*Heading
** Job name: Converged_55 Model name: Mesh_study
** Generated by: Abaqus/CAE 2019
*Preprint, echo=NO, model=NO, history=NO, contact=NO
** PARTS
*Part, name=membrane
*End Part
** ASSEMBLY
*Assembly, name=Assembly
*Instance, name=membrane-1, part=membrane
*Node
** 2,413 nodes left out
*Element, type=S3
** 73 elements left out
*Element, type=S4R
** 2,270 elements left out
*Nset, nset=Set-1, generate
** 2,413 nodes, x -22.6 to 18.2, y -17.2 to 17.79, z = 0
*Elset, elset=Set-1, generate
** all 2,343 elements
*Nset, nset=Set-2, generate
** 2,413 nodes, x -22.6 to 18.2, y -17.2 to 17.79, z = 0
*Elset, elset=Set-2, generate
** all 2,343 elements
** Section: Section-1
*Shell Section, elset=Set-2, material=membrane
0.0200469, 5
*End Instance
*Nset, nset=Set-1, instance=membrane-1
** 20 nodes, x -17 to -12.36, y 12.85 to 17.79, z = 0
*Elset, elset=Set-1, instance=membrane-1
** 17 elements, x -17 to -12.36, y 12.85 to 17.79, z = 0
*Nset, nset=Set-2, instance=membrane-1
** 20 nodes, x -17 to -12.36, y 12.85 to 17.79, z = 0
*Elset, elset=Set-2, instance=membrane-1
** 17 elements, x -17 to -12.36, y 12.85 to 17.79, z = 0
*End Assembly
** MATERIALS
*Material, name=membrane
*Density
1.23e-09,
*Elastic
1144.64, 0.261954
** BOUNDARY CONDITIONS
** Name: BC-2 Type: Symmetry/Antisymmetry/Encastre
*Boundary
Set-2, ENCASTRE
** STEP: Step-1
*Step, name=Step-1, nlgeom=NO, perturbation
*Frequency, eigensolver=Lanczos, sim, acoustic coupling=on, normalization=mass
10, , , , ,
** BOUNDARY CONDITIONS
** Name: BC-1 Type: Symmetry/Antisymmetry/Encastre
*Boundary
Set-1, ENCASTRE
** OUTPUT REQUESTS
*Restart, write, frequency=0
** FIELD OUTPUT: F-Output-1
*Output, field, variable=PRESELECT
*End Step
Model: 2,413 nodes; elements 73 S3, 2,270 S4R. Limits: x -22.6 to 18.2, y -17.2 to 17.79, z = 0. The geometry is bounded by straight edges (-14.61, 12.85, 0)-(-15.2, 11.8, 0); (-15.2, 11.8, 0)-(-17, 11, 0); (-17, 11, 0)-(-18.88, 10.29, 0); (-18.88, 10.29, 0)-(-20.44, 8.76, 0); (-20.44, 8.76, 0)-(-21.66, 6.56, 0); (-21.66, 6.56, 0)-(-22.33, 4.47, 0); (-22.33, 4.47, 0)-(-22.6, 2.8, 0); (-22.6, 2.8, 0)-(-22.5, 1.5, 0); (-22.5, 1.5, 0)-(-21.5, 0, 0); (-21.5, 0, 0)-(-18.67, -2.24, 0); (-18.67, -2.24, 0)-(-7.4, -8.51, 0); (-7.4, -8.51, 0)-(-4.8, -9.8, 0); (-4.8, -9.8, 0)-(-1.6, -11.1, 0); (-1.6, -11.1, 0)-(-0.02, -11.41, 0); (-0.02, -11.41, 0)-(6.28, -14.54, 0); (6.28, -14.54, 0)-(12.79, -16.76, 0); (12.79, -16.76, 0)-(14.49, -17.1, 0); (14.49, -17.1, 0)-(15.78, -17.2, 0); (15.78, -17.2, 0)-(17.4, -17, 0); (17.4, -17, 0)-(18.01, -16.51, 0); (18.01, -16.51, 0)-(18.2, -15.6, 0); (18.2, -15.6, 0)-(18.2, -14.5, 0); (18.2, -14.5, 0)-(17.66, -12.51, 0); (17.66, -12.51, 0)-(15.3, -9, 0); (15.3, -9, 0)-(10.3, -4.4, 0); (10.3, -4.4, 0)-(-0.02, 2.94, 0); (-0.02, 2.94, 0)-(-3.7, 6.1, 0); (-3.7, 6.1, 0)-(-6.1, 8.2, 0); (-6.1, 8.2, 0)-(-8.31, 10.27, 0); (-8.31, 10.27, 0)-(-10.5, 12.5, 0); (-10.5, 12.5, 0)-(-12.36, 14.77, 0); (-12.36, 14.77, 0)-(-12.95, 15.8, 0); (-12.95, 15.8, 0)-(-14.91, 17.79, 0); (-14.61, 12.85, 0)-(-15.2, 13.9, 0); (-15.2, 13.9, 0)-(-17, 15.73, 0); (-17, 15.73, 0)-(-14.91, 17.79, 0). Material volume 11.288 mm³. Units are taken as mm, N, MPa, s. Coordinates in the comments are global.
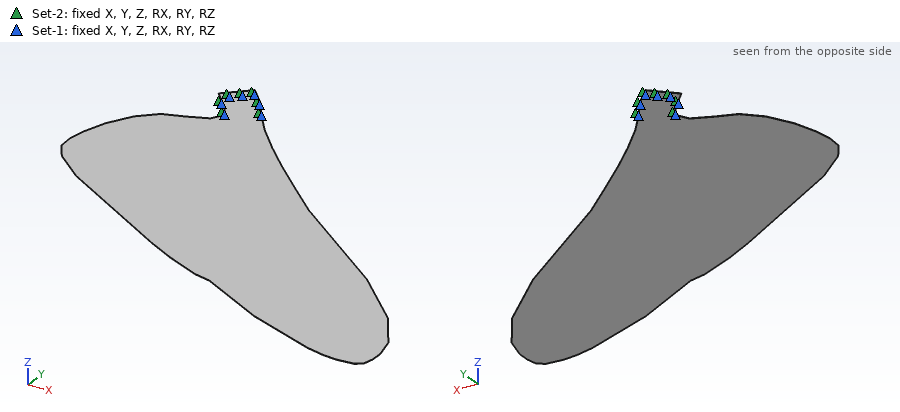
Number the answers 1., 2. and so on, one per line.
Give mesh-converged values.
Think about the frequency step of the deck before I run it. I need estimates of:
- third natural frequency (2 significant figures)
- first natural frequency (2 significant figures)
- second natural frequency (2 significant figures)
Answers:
1. 13 Hz
2. 1.6 Hz
3. 6.7 Hz
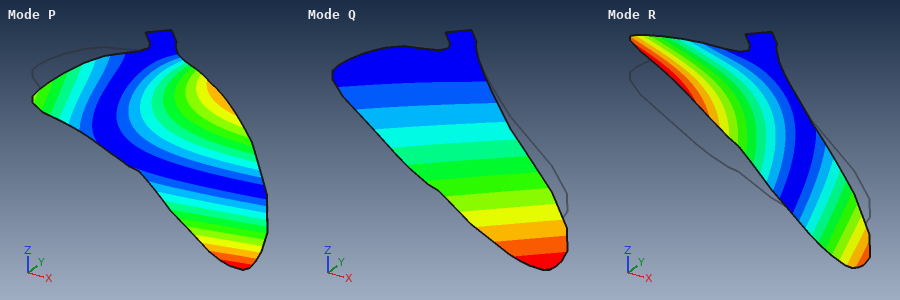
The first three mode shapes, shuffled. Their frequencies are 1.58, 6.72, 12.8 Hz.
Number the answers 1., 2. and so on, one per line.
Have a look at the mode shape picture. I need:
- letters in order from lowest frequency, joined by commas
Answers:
1. Q, R, P
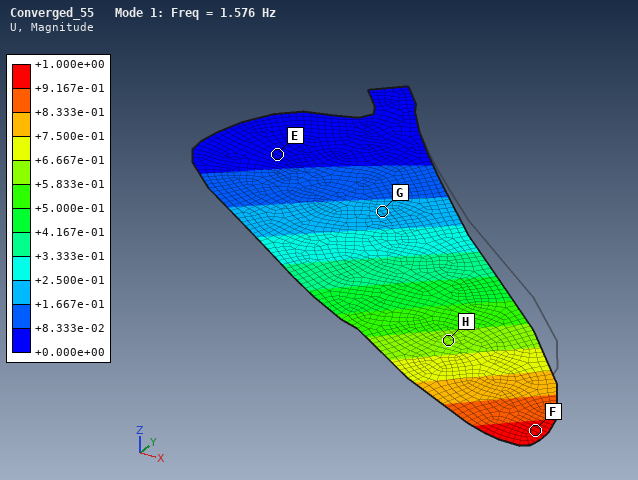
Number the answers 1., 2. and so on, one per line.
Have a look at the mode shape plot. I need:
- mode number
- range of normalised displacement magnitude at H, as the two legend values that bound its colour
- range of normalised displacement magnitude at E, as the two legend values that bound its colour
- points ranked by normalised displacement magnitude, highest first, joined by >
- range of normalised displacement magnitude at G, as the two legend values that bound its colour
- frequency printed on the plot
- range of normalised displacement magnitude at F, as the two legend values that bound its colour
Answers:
1. 1
2. +5.833e-01 to +6.667e-01
3. +0.000e+00 to +8.333e-02
4. F > H > G > E
5. +1.667e-01 to +2.500e-01
6. 1.576 Hz
7. +9.167e-01 to +1.000e+00
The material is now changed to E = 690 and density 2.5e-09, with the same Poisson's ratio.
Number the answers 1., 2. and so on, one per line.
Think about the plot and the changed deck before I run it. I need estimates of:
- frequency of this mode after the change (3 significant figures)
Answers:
1. 0.858 Hz
